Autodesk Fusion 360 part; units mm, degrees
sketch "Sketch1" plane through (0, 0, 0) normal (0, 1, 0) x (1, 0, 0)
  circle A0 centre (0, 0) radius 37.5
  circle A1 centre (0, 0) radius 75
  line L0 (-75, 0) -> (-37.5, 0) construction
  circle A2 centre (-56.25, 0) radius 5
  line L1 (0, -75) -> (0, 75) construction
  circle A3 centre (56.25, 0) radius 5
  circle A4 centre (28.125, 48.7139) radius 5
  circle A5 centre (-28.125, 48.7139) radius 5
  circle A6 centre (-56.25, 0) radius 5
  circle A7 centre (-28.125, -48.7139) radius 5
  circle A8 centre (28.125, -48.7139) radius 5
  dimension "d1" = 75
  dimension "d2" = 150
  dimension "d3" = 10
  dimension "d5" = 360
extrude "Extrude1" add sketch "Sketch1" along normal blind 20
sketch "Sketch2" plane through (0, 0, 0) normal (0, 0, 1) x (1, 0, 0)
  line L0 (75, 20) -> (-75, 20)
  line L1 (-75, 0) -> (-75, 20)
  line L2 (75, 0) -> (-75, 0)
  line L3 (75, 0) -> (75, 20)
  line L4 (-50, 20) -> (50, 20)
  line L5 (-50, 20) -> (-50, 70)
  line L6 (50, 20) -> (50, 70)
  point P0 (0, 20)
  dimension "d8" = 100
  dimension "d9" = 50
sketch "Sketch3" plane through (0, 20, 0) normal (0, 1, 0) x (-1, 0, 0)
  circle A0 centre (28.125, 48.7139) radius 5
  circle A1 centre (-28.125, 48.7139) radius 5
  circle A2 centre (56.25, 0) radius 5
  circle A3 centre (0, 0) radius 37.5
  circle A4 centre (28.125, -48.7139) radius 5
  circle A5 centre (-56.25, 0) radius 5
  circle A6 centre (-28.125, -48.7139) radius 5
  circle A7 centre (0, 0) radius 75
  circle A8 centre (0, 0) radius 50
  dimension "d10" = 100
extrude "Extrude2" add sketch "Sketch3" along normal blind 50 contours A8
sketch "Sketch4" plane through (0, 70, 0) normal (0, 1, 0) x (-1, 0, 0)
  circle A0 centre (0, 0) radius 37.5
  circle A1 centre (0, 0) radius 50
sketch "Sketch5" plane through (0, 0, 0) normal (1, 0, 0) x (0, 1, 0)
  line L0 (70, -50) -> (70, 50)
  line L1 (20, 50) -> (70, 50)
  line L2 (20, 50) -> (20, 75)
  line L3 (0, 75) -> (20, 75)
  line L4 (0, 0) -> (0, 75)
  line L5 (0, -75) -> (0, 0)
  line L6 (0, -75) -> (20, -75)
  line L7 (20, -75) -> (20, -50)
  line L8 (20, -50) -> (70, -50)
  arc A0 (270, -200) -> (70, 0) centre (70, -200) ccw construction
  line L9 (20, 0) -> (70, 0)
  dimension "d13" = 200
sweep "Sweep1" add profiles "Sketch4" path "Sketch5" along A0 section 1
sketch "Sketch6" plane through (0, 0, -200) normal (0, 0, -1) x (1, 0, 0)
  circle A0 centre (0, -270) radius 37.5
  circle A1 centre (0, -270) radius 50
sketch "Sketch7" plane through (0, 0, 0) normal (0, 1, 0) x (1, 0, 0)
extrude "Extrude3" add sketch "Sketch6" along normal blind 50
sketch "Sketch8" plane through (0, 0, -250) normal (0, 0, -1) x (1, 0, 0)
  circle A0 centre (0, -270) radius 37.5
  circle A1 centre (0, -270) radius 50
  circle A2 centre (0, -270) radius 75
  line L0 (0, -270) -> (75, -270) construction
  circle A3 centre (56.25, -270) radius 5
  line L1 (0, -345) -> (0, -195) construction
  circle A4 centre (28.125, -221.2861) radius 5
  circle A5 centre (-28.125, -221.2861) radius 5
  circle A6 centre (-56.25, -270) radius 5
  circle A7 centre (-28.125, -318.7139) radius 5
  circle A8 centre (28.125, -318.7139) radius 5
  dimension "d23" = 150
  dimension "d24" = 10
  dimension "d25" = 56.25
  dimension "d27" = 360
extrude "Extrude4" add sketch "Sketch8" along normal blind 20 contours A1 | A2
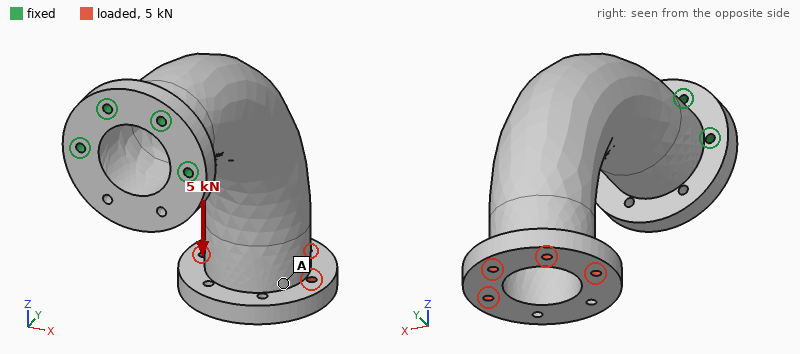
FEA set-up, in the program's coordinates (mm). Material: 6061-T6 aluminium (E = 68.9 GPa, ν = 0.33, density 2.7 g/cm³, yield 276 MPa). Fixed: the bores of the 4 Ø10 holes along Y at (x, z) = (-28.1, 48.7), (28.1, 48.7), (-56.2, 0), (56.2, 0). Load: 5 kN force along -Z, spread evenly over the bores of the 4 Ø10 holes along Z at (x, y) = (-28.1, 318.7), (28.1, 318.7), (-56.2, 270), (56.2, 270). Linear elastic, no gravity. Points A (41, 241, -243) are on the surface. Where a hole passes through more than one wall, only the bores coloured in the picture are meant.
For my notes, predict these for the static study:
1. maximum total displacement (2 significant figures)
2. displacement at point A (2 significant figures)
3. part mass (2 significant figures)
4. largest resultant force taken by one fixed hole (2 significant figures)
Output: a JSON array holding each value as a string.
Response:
["0.77 mm", "0.59 mm", "5.2 kg", "13 kN"]
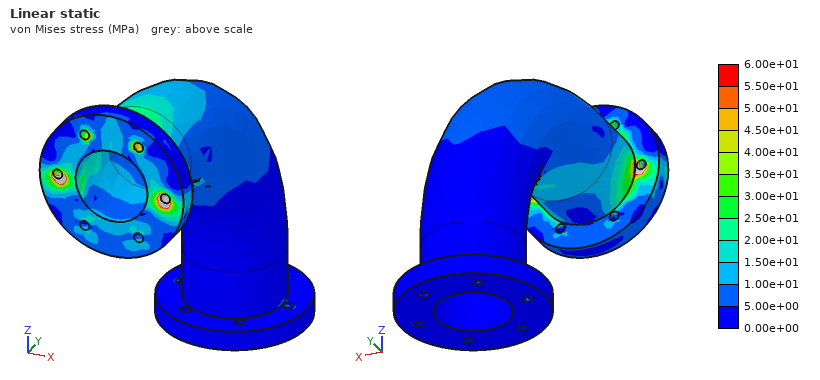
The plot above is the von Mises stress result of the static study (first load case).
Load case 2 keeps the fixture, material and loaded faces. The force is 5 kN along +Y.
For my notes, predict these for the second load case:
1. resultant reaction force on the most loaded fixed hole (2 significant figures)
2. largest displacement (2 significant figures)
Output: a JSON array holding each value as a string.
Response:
["14 kN", "0.95 mm"]
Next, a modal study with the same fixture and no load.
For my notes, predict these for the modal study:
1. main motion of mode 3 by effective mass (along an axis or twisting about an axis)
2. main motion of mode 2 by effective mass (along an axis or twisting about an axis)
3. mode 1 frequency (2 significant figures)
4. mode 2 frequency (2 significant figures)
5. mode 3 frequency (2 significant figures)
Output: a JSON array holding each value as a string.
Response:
["along Z", "along X", "260 Hz", "340 Hz", "1000 Hz"]
